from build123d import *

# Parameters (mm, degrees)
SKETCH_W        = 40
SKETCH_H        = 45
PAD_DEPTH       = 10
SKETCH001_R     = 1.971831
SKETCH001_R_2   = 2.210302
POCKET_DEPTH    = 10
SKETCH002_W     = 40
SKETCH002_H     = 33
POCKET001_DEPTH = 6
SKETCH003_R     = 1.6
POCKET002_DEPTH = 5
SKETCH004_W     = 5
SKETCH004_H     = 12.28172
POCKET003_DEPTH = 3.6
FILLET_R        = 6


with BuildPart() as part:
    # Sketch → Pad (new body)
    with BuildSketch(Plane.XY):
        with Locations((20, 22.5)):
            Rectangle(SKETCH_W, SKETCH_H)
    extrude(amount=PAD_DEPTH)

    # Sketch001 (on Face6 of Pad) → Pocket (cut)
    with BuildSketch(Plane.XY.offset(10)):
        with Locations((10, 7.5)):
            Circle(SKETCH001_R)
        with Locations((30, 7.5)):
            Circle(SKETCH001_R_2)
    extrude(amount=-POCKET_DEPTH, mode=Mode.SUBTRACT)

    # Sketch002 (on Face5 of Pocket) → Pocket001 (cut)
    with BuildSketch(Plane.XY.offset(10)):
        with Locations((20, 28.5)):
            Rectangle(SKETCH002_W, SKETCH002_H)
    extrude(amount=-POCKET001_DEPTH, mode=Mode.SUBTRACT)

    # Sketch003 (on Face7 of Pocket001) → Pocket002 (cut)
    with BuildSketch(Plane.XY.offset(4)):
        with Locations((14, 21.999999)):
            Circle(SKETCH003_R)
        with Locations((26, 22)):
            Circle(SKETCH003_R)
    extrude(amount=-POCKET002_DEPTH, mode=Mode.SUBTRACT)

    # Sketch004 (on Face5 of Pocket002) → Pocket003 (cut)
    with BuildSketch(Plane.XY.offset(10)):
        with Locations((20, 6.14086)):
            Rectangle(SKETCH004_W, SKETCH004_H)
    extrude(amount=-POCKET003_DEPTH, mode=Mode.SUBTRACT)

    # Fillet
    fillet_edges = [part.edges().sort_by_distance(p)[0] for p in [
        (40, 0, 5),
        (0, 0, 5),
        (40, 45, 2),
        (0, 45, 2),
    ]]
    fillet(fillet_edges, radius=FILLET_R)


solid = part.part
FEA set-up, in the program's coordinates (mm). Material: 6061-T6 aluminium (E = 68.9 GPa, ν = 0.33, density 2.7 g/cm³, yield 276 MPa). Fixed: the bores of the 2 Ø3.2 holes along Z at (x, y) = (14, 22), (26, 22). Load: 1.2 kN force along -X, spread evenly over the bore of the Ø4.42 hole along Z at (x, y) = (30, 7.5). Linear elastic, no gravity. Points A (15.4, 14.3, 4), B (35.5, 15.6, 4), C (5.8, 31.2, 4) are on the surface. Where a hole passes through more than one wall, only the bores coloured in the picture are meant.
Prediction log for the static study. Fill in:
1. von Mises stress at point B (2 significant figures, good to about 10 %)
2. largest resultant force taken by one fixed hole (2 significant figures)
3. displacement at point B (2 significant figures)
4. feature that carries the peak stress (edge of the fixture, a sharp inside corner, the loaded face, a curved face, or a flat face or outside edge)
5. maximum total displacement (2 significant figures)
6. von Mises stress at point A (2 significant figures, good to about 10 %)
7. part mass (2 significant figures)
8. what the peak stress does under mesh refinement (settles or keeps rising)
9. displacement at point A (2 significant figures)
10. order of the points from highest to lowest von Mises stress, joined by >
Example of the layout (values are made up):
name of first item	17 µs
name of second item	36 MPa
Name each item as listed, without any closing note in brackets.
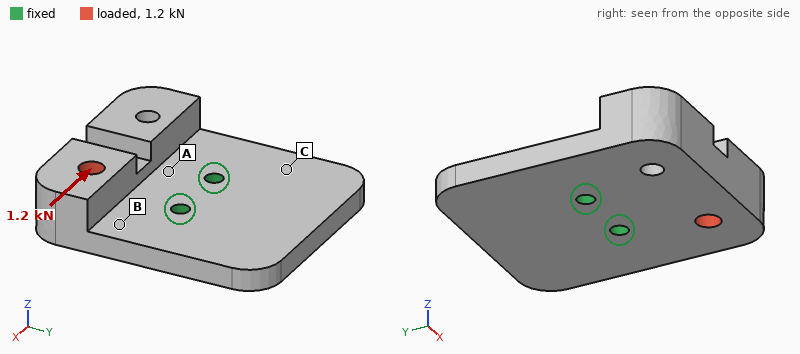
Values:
von Mises stress at point B	17 MPa
largest resultant force taken by one fixed hole	1.4 kN
displacement at point B	14 µm
feature that carries the peak stress	edge of the fixture
maximum total displacement	30 µm
von Mises stress at point A	33 MPa
part mass	25 g
what the peak stress does under mesh refinement	keeps rising
displacement at point A	6.7 µm
order of the points from highest to lowest von Mises stress, joined by >	A > B > C
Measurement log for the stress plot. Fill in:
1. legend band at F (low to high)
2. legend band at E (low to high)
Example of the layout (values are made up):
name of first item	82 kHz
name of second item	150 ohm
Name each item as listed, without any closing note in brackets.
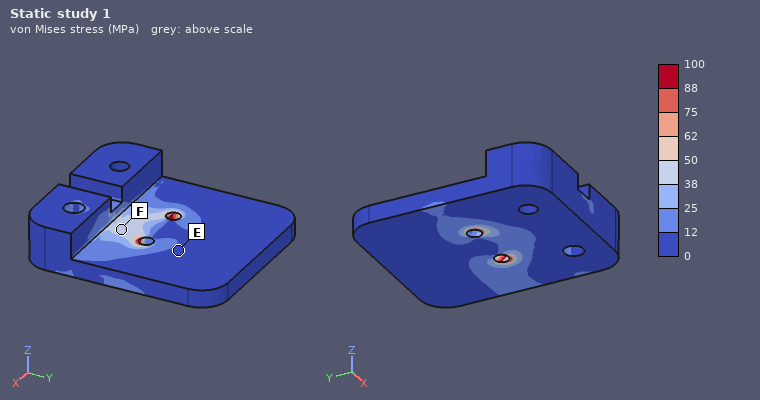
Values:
legend band at F	38 to 50 MPa
legend band at E	0 to 12 MPa
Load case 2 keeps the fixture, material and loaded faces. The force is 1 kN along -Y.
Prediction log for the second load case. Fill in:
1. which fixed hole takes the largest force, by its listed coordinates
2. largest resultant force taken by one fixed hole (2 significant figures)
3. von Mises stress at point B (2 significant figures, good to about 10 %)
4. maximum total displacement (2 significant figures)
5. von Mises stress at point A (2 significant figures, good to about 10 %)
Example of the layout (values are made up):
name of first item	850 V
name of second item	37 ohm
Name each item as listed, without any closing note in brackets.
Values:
which fixed hole takes the largest force, by its listed coordinates	(26, 22)
largest resultant force taken by one fixed hole	1.2 kN
von Mises stress at point B	36 MPa
maximum total displacement	57 µm
von Mises stress at point A	25 MPa
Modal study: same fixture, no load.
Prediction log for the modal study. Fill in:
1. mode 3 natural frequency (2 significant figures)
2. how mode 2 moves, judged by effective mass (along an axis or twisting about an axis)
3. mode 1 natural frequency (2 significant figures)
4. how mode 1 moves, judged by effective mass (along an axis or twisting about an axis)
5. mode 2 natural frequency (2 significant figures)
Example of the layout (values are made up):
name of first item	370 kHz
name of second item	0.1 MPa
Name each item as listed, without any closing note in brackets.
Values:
mode 3 natural frequency	7100 Hz
how mode 2 moves, judged by effective mass	along Z
mode 1 natural frequency	4000 Hz
how mode 1 moves, judged by effective mass	along Z
mode 2 natural frequency	6100 Hz
